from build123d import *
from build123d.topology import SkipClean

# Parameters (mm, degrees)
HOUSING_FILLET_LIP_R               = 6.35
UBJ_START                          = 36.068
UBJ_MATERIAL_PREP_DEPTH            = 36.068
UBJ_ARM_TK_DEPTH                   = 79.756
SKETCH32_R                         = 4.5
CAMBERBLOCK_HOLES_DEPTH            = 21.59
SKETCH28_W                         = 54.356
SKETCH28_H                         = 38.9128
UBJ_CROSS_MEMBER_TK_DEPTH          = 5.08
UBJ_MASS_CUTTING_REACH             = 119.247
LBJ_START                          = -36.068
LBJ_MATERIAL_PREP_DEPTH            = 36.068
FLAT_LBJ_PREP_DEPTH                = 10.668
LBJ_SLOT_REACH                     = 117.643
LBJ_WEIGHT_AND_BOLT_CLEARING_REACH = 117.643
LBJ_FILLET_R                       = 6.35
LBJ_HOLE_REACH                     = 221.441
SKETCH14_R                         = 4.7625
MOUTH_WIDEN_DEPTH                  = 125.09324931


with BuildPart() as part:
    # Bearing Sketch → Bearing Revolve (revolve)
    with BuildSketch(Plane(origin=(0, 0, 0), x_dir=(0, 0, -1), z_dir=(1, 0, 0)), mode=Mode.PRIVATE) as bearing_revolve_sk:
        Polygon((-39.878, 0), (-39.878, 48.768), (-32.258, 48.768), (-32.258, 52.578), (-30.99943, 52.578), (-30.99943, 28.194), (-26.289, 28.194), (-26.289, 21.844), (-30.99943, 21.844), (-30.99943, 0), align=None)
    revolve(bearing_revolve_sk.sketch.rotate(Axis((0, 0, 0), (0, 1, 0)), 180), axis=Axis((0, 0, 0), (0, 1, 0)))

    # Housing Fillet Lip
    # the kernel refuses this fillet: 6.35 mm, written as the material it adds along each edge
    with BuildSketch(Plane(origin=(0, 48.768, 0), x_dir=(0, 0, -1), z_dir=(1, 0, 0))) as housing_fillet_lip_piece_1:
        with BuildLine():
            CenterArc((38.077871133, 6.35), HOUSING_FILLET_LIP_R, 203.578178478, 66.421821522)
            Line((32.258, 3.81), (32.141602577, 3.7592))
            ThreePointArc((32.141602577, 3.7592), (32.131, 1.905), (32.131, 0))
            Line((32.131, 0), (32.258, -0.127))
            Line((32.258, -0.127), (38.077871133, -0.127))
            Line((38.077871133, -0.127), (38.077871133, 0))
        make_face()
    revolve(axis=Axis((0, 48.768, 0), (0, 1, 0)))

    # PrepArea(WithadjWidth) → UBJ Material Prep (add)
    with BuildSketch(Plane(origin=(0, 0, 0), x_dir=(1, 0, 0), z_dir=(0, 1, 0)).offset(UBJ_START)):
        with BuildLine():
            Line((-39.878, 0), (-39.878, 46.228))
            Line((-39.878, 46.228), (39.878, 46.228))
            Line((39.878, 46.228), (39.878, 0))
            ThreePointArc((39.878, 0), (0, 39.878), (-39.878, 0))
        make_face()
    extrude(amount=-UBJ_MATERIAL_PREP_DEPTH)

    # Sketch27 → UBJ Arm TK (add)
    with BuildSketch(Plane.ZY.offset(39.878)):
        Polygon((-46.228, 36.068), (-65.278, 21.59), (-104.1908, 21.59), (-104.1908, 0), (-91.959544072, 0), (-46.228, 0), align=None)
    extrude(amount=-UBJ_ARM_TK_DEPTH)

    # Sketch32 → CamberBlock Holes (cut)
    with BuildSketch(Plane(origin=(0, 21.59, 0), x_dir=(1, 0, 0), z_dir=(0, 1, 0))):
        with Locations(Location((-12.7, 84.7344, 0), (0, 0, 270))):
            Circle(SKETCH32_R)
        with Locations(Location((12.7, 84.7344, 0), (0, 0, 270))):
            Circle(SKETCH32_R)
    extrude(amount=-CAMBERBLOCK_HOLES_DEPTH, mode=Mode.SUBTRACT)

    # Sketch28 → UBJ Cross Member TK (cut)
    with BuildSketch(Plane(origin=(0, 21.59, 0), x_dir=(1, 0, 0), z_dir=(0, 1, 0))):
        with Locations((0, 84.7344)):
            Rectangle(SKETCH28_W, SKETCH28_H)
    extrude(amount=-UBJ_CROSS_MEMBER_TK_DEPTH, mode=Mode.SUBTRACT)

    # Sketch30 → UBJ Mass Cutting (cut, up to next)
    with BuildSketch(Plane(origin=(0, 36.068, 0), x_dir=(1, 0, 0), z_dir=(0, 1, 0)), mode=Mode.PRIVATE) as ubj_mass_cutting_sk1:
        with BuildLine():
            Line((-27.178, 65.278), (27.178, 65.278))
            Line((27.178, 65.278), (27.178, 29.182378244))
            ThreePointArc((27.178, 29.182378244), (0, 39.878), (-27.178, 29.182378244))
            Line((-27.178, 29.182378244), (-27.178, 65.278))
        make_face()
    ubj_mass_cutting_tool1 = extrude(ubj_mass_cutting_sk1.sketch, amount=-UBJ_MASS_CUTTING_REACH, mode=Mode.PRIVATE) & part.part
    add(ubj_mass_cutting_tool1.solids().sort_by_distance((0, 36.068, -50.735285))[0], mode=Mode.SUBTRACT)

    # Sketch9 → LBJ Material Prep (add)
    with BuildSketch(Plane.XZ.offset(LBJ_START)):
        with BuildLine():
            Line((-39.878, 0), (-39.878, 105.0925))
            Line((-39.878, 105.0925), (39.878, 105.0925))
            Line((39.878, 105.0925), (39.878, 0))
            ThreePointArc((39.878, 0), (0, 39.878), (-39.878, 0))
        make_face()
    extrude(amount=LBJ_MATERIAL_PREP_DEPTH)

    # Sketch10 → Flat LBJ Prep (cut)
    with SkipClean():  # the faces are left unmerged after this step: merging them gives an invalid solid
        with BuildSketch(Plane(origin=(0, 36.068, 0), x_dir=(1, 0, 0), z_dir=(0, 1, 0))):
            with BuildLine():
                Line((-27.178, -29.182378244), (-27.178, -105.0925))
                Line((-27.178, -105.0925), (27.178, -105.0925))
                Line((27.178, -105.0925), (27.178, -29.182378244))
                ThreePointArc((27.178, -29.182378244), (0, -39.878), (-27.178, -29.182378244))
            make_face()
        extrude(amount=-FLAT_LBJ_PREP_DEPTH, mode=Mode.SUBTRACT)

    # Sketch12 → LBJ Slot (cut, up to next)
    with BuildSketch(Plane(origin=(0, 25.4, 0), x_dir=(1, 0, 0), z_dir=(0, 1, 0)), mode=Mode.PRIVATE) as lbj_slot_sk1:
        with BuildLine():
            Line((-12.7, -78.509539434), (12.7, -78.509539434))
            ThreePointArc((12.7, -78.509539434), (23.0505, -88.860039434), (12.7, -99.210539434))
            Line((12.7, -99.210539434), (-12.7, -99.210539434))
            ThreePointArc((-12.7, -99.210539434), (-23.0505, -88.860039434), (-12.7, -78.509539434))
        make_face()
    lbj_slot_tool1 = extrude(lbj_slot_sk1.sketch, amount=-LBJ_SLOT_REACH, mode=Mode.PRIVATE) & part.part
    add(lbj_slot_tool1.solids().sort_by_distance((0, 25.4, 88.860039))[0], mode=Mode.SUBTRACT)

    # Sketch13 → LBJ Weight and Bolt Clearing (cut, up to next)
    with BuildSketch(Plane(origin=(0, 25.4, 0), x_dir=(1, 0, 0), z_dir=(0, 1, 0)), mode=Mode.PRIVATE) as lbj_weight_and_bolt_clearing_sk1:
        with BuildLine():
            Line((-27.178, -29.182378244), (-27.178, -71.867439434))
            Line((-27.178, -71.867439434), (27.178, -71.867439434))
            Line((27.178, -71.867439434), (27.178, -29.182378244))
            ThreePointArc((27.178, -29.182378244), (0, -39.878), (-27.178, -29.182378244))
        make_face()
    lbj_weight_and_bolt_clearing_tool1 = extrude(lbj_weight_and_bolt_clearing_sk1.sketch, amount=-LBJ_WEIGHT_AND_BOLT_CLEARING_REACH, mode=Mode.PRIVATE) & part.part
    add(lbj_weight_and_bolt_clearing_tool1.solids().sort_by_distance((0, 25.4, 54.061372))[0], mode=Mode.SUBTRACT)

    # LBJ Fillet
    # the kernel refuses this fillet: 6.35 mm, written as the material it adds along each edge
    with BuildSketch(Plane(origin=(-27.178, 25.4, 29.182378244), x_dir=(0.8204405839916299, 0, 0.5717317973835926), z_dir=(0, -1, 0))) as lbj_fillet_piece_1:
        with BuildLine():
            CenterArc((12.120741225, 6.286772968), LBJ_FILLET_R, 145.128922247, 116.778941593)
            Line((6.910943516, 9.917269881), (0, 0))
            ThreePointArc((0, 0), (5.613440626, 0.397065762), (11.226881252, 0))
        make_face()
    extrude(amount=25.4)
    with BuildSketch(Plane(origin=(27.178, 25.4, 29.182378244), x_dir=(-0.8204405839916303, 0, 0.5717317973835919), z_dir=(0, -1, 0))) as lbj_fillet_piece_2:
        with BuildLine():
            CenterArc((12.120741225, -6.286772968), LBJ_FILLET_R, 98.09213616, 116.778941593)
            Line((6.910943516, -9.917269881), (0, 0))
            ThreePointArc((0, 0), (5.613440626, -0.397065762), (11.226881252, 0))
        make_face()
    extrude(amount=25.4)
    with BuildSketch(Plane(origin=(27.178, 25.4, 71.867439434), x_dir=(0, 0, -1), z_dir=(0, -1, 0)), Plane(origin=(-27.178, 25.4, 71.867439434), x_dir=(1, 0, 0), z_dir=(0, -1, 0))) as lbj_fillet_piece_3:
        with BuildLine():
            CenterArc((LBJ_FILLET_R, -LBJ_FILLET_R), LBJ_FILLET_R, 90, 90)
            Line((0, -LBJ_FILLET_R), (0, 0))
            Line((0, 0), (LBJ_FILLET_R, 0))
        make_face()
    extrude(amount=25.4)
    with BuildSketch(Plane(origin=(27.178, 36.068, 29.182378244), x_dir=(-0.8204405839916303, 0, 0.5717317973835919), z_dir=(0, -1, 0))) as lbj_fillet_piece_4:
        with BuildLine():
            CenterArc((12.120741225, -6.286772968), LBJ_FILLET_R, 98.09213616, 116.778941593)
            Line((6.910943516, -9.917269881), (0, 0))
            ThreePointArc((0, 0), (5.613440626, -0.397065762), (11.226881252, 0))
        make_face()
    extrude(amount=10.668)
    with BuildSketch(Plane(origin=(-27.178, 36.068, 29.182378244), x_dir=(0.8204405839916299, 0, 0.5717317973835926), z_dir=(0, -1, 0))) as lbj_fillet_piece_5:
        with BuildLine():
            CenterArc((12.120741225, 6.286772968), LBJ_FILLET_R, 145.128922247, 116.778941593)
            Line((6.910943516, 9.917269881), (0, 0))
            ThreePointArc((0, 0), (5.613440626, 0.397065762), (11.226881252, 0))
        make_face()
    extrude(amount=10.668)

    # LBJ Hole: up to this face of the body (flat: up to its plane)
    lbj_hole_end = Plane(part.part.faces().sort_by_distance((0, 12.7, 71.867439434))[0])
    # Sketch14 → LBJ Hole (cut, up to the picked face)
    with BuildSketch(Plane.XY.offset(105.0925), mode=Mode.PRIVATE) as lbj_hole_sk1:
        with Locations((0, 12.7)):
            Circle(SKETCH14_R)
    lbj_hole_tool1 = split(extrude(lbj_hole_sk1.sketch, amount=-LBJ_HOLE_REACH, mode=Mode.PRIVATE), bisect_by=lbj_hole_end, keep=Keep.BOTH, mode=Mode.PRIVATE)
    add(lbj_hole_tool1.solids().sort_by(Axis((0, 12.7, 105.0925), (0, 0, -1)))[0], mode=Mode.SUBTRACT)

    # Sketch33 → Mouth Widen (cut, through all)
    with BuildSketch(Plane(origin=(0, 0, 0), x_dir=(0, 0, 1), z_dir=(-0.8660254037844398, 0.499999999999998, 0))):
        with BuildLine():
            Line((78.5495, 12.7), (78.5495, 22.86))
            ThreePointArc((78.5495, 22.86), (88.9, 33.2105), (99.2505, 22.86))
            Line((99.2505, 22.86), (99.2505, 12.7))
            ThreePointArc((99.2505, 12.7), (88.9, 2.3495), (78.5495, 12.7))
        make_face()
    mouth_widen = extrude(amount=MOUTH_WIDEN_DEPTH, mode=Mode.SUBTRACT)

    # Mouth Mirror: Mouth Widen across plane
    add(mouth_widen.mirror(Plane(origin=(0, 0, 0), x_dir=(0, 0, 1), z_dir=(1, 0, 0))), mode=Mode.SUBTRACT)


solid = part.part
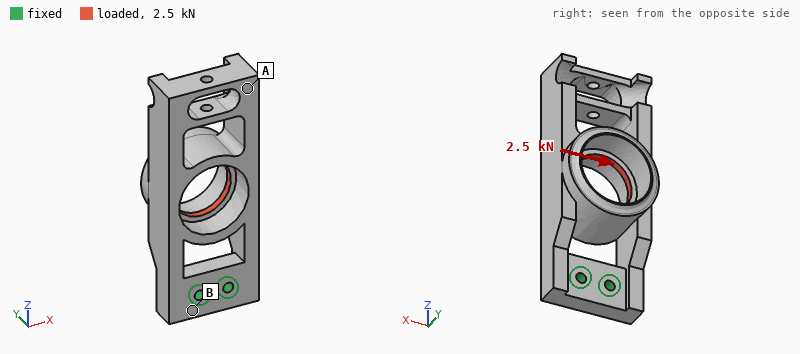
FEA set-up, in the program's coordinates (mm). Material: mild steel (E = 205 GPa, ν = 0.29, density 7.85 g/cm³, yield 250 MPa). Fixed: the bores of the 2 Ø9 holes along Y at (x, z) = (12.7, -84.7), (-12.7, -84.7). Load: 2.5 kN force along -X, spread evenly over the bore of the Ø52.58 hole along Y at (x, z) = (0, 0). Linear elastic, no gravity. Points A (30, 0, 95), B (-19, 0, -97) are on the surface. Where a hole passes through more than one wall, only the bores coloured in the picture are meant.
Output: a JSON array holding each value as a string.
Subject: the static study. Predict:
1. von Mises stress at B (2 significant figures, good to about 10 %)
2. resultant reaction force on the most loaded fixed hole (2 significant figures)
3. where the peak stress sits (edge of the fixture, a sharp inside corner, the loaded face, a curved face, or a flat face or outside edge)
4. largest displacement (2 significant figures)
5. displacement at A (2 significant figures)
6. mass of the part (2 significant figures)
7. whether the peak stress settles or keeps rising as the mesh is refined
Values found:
["12 MPa", "5.7 kN", "edge of the fixture", "76 µm", "73 µm", "2.3 kg", "keeps rising"]
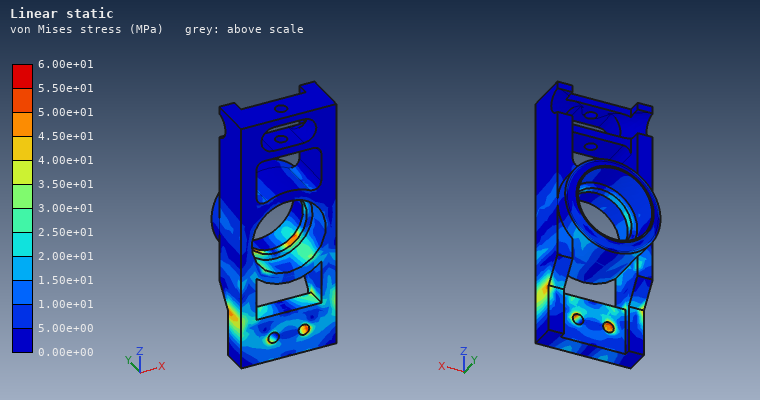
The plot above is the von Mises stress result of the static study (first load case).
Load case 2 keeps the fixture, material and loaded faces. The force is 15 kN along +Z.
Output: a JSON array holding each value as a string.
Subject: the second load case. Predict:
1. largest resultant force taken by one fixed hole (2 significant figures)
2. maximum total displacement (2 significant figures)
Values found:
["7.5 kN", "0.35 mm"]
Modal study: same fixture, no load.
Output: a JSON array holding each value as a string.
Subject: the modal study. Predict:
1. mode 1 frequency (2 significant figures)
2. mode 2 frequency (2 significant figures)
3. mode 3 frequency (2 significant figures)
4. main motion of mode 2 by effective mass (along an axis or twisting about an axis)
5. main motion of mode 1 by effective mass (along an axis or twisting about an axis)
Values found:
["370 Hz", "680 Hz", "1200 Hz", "along X", "along Y"]
